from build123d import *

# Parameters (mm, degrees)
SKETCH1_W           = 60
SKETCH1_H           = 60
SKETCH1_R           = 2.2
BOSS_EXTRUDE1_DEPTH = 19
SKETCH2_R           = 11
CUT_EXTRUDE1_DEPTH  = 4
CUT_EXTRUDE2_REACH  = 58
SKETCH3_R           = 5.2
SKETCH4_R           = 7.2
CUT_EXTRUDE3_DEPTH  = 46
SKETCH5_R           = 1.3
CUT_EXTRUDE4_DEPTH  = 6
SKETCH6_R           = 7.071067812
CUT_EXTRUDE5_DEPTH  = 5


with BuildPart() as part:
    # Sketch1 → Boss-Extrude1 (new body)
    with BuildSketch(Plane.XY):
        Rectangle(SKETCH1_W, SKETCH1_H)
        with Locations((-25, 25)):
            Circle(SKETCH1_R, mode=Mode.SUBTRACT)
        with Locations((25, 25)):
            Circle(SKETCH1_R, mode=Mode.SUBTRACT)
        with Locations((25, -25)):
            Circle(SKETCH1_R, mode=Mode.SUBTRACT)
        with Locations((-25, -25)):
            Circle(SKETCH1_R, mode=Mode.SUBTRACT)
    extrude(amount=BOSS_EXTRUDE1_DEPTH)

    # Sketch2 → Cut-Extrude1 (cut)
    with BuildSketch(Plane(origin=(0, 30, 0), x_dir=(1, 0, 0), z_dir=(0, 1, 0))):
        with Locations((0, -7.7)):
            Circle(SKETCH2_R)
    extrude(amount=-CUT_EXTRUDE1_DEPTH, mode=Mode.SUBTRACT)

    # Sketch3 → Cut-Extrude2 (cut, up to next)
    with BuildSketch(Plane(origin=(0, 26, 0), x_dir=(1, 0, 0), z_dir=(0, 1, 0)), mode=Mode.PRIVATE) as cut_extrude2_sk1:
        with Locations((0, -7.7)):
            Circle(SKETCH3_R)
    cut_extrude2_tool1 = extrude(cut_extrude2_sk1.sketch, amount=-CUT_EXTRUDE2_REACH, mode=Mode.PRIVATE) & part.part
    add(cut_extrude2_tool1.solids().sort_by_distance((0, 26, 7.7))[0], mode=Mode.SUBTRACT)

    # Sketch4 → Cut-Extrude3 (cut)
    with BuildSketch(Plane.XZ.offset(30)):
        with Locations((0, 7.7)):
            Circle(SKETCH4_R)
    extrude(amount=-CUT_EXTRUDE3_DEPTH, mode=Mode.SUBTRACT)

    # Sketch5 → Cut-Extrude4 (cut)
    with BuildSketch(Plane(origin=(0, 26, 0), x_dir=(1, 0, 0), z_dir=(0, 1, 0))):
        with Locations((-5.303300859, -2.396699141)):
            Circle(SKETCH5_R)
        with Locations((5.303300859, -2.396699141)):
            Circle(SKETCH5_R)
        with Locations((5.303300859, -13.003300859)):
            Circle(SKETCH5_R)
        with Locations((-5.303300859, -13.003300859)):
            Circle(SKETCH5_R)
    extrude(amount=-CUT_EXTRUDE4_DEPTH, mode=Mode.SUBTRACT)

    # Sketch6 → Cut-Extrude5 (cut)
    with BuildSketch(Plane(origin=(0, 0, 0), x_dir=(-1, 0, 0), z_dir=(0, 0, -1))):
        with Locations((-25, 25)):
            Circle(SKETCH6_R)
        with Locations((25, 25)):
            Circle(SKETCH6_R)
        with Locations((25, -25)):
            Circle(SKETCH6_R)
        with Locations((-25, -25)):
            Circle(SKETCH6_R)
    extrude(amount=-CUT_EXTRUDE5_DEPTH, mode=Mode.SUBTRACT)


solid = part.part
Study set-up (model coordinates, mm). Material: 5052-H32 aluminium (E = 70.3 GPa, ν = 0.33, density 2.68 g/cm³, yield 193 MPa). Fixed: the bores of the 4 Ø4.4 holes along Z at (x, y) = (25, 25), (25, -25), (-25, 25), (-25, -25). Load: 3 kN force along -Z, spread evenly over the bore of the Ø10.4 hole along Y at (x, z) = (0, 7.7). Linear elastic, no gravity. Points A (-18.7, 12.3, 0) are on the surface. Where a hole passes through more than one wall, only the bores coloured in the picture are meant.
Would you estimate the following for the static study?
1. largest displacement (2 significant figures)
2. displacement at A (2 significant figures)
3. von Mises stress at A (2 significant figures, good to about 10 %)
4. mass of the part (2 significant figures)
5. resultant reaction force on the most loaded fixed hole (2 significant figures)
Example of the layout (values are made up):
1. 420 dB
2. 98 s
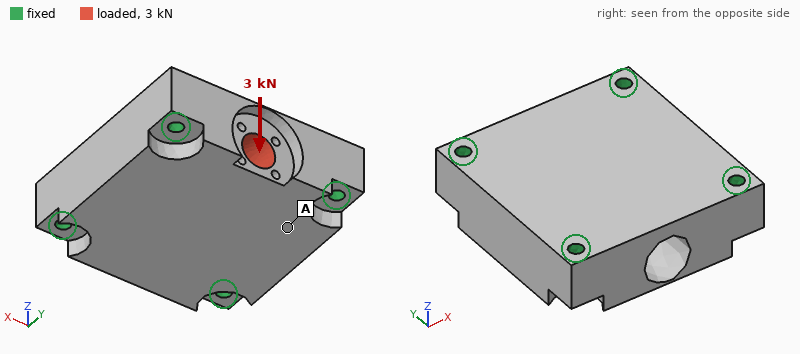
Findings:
1. 14 µm
2. 3.7 µm
3. 5.5 MPa
4. 150 g
5. 1.4 kN
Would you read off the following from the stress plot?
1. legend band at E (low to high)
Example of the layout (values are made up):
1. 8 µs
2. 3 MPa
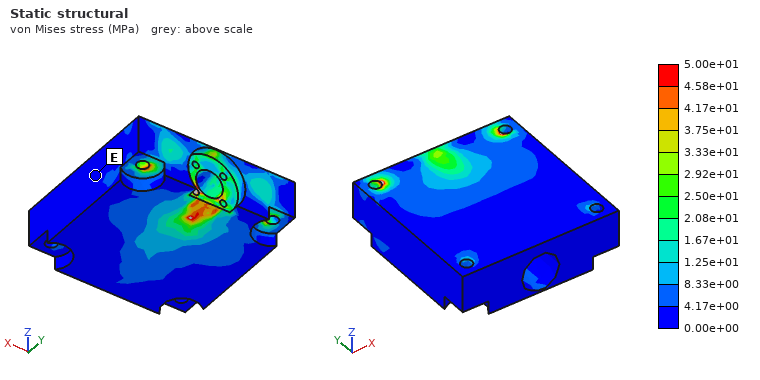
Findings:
1. 0.00e+00 to 4.17e+00 MPa
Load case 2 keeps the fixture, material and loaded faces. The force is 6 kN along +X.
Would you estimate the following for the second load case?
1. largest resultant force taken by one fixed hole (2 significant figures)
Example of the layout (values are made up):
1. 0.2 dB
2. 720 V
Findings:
1. 2.6 kN
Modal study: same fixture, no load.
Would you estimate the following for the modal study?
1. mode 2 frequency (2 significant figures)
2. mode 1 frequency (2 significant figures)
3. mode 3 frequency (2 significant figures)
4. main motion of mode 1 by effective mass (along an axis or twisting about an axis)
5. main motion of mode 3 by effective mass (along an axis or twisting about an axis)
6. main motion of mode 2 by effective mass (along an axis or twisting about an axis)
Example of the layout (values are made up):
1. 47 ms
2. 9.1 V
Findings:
1. 21 kHz
2. 15 kHz
3. 21 kHz
4. along Z
5. along X
6. twisting about Y
